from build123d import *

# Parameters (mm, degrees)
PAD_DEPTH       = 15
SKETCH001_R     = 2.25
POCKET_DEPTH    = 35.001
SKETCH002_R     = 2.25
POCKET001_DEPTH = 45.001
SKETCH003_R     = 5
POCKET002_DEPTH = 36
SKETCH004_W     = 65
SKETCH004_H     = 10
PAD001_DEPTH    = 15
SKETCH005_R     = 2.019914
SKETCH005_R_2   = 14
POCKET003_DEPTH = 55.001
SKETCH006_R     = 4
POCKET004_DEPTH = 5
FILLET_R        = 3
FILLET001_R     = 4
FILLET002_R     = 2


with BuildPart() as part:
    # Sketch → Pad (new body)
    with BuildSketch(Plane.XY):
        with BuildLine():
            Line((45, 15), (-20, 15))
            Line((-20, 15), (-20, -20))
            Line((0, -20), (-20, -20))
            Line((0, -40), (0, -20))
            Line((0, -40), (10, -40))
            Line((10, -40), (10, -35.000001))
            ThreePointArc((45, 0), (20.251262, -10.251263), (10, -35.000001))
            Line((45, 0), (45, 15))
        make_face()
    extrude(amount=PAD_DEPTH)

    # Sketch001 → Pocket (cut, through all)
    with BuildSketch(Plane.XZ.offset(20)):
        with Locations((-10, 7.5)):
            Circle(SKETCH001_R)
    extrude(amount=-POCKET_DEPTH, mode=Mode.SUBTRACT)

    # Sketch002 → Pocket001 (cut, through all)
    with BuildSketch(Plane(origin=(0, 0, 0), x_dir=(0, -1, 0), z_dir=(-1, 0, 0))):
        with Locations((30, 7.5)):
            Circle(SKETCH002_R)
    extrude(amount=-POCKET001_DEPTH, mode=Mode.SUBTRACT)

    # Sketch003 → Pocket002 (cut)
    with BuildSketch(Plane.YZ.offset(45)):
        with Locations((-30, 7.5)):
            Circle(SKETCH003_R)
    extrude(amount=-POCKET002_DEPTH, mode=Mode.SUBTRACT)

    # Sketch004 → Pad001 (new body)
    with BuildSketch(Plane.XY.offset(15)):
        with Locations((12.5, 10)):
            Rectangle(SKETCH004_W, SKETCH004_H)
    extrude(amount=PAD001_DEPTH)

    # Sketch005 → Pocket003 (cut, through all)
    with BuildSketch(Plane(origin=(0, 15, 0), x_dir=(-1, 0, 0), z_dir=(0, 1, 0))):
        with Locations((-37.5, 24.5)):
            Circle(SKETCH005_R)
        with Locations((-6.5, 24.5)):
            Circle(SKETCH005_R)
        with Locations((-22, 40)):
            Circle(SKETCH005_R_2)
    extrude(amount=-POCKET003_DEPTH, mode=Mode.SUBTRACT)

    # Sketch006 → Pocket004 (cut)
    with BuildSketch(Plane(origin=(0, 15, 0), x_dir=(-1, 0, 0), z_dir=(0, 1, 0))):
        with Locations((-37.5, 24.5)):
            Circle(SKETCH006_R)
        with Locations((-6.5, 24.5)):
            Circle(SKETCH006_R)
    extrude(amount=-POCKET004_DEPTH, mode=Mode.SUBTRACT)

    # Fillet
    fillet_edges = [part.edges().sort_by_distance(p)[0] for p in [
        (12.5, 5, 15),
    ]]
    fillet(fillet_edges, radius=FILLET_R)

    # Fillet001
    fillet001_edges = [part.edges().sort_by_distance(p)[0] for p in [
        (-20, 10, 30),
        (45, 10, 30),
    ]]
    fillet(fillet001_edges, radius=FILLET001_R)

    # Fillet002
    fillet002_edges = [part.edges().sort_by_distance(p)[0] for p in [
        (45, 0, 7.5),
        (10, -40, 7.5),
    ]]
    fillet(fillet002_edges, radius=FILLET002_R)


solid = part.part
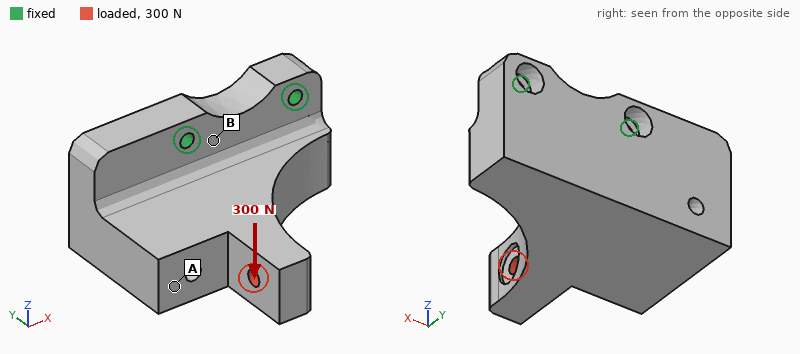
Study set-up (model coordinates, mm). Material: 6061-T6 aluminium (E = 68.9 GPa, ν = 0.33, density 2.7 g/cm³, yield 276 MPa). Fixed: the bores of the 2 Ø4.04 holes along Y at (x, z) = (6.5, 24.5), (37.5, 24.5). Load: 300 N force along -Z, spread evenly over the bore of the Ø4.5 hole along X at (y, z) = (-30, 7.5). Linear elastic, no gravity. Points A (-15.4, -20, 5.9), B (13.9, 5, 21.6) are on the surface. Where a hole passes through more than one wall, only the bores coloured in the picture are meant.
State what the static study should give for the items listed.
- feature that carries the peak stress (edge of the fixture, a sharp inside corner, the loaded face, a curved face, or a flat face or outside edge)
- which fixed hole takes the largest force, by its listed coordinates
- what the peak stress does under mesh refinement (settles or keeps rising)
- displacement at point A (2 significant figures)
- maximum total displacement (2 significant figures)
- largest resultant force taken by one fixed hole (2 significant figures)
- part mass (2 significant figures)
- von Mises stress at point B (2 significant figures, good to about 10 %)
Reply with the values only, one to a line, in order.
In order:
edge of the fixture
(6.5, 24.5)
keeps rising
55 µm
96 µm
320 N
100 g
13 MPa
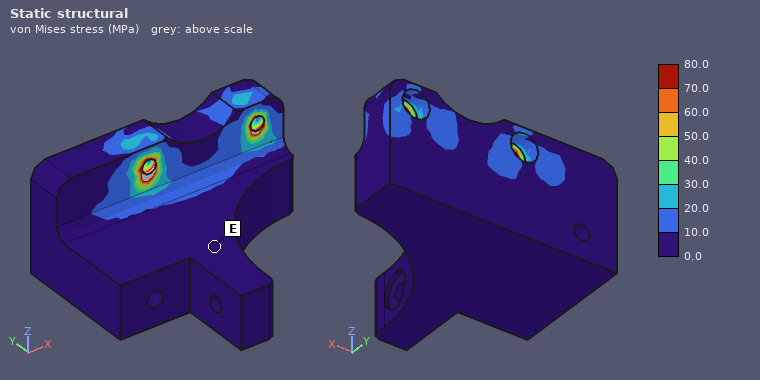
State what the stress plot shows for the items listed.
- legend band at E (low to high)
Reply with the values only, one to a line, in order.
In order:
0.0 to 10.0 MPa
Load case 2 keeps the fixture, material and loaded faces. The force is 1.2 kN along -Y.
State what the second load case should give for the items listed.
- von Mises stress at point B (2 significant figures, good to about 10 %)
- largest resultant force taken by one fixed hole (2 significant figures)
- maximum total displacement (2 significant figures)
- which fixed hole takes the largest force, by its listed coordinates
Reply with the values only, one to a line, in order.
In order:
16 MPa
1.2 kN
0.14 mm
(6.5, 24.5)
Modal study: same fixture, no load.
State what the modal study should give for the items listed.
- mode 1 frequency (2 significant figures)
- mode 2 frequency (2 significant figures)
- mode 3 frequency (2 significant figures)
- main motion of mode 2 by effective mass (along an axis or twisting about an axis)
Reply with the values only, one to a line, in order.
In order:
2000 Hz
4500 Hz
8100 Hz
along X
